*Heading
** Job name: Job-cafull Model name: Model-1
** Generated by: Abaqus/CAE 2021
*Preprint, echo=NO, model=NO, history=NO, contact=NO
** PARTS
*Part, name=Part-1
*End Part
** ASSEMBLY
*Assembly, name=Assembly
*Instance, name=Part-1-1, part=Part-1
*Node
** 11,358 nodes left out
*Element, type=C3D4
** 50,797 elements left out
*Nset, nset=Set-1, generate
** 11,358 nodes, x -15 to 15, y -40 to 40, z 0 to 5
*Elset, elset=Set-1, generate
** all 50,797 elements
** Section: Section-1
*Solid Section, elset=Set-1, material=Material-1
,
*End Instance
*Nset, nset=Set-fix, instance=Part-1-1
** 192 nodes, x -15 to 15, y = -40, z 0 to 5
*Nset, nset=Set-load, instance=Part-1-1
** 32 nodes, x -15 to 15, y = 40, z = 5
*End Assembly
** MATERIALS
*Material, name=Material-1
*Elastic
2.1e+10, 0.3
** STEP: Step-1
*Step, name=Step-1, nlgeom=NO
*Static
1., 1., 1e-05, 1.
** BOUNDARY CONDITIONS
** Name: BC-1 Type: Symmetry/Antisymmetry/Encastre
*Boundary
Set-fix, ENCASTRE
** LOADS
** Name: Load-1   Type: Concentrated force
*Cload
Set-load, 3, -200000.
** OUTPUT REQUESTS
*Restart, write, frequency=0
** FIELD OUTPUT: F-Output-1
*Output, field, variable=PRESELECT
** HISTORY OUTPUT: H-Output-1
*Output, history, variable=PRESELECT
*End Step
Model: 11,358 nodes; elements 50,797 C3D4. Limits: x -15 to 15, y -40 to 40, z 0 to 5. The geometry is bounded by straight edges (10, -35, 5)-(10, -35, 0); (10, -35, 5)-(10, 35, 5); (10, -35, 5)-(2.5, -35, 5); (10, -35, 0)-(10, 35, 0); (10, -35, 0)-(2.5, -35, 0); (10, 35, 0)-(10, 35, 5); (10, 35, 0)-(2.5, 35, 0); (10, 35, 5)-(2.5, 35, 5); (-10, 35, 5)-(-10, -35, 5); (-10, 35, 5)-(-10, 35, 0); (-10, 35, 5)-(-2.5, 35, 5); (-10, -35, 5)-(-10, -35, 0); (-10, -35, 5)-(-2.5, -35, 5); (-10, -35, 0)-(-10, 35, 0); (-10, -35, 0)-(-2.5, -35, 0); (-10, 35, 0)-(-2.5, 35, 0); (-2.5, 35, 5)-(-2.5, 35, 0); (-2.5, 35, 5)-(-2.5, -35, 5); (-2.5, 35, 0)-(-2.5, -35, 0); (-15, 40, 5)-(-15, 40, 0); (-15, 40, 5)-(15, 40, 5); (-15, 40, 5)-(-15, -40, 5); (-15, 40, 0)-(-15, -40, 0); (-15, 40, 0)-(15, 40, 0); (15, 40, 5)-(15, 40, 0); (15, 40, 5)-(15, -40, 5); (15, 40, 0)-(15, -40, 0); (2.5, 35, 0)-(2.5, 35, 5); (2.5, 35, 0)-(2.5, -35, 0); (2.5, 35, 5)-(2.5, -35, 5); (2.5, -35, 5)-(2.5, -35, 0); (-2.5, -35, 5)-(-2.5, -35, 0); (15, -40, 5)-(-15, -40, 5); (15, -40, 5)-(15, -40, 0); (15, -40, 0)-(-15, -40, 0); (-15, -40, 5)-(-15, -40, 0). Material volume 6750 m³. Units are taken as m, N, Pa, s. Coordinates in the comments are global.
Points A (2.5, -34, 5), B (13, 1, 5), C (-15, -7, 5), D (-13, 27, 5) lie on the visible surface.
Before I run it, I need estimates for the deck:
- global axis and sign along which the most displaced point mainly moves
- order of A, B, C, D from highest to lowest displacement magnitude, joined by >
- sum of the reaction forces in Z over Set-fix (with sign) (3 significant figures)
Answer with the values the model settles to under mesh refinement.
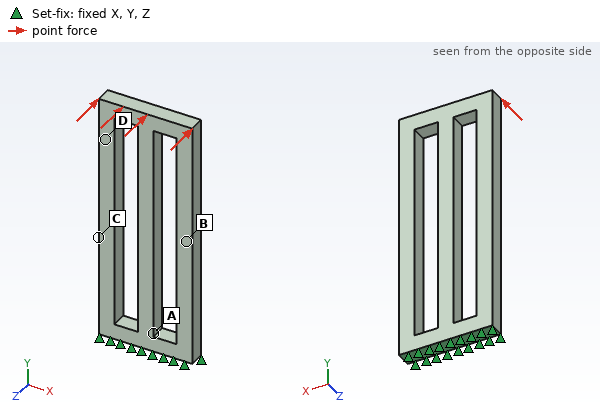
-Z
D > B > C > A
6.40e+06 N
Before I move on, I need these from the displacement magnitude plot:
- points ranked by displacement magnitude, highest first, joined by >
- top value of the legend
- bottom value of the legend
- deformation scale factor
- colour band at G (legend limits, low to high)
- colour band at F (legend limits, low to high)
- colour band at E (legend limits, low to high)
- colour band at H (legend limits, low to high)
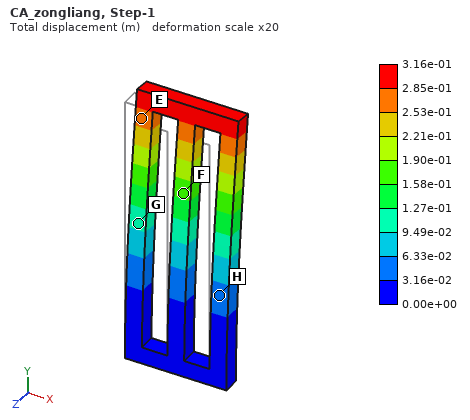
E > F > G > H
3.16e-01 m
0.00e+00 m
20
9.49e-02 to 1.27e-01 m
1.58e-01 to 1.90e-01 m
2.53e-01 to 2.85e-01 m
3.16e-02 to 6.33e-02 m
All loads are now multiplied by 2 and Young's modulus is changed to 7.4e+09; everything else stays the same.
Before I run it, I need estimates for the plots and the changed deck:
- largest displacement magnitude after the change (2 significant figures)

1.8 m
